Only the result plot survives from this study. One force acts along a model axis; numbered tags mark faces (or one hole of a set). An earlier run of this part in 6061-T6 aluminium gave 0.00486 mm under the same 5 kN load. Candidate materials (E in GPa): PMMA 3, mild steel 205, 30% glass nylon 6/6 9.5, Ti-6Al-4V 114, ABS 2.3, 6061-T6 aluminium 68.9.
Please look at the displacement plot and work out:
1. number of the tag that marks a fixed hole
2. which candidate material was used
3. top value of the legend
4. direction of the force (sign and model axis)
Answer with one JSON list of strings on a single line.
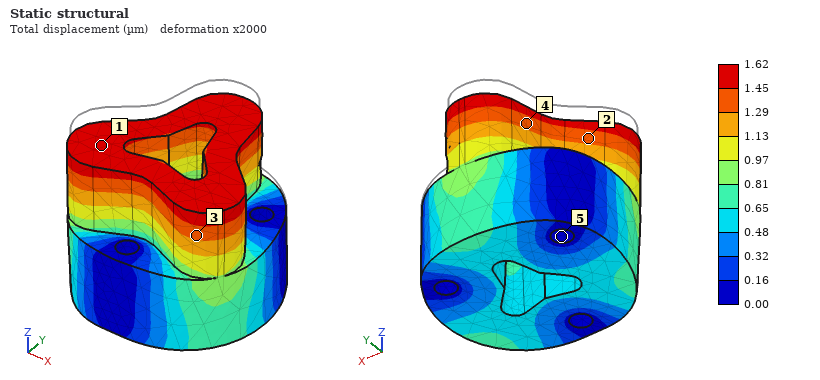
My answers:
["5", "mild steel", "1.62 µm", "-Z"]
